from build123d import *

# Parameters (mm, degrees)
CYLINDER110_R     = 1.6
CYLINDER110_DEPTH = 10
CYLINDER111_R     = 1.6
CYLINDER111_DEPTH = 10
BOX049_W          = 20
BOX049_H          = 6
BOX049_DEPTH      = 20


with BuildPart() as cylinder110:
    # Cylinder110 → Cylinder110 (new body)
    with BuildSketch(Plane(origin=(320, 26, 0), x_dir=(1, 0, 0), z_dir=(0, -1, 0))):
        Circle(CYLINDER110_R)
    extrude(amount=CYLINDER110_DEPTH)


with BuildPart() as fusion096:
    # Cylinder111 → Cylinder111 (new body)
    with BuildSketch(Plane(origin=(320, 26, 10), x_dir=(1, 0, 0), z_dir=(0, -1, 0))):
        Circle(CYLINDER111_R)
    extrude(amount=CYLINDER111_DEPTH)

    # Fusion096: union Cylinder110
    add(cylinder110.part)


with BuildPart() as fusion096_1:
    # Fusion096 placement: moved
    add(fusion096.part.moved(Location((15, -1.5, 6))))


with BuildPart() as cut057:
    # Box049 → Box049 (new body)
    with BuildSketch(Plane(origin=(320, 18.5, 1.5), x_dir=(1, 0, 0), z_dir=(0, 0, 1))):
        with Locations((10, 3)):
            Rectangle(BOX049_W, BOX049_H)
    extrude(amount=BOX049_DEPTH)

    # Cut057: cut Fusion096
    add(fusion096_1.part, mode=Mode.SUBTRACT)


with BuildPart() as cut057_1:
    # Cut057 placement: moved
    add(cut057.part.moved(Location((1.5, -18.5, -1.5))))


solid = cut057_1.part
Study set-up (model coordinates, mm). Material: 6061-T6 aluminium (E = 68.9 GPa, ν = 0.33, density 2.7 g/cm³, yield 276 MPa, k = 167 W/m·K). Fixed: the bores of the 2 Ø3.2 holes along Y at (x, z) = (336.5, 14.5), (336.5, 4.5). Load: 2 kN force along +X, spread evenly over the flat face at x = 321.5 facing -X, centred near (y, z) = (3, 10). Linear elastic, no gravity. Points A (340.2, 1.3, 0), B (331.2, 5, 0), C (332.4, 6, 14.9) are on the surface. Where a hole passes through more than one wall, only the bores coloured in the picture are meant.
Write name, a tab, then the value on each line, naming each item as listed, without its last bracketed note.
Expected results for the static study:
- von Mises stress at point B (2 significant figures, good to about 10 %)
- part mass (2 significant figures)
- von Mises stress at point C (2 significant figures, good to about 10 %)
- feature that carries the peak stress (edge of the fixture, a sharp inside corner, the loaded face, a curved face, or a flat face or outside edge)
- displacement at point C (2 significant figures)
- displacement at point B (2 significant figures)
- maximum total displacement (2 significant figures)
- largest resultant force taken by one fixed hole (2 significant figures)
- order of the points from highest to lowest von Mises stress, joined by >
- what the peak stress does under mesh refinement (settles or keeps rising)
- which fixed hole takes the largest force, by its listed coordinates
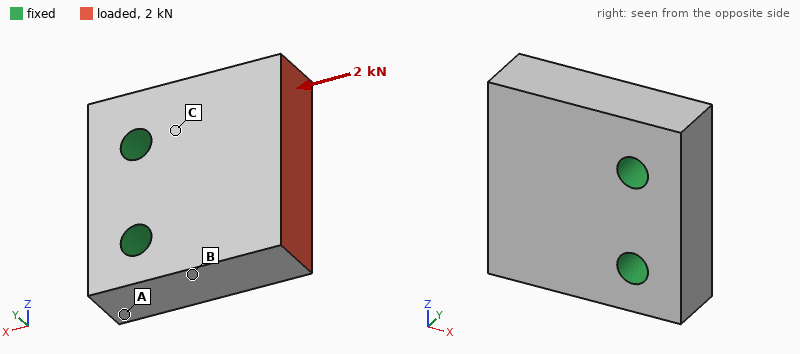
von Mises stress at point B	12 MPa
part mass	6.2 g
von Mises stress at point C	22 MPa
feature that carries the peak stress	edge of the fixture
displacement at point C	1.1 µm
displacement at point B	1.6 µm
maximum total displacement	4.3 µm
largest resultant force taken by one fixed hole	1.1 kN
order of the points from highest to lowest von Mises stress, joined by >	C > B > A
what the peak stress does under mesh refinement	keeps rising
which fixed hole takes the largest force, by its listed coordinates	(336.5, 14.5)
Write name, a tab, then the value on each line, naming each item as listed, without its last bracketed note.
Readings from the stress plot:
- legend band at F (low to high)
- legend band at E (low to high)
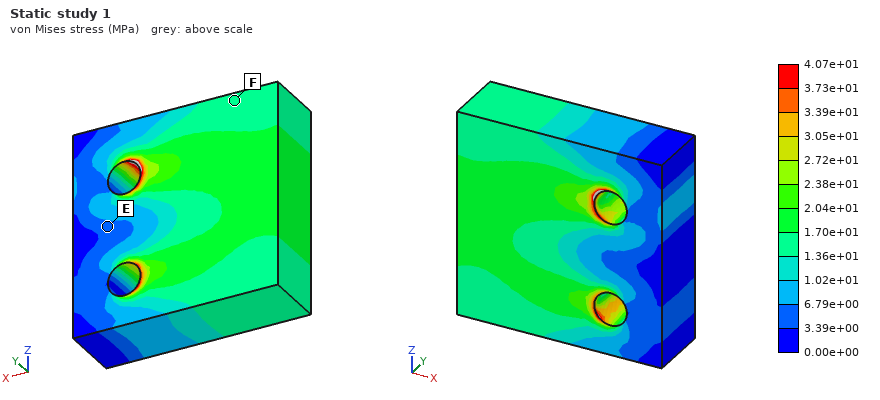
legend band at F	1.36e+01 to 1.70e+01 MPa
legend band at E	3.39e+00 to 6.79e+00 MPa
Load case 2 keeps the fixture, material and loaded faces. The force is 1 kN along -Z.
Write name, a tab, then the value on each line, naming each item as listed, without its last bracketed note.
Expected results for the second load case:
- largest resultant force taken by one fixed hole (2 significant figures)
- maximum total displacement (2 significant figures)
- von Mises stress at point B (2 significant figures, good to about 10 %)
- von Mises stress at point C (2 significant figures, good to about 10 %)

largest resultant force taken by one fixed hole	1.3 kN
maximum total displacement	14 µm
von Mises stress at point B	22 MPa
von Mises stress at point C	24 MPa
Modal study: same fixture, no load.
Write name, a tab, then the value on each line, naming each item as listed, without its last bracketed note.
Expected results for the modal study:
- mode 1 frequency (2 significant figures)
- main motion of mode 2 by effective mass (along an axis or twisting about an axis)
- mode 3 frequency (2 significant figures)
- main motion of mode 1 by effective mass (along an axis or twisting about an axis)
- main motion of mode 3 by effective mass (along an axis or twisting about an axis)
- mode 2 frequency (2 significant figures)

mode 1 frequency	20 kHz
main motion of mode 2 by effective mass	twisting about X
mode 3 frequency	36 kHz
main motion of mode 1 by effective mass	along Y
main motion of mode 3 by effective mass	along Z
mode 2 frequency	33 kHz
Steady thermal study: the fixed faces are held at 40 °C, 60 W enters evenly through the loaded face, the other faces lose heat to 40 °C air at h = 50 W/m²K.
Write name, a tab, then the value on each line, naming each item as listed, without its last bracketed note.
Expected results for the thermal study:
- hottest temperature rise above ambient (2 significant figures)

hottest temperature rise above ambient	43 K
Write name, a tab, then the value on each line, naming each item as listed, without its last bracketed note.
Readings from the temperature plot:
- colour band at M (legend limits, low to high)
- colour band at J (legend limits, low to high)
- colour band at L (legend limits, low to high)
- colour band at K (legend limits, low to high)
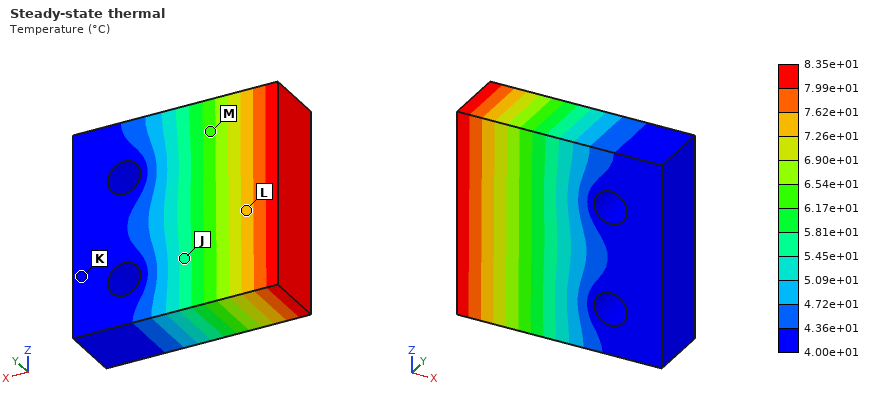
colour band at M	6.17e+01 to 6.54e+01 °C
colour band at J	5.45e+01 to 5.81e+01 °C
colour band at L	7.26e+01 to 7.62e+01 °C
colour band at K	4.00e+01 to 4.36e+01 °C
